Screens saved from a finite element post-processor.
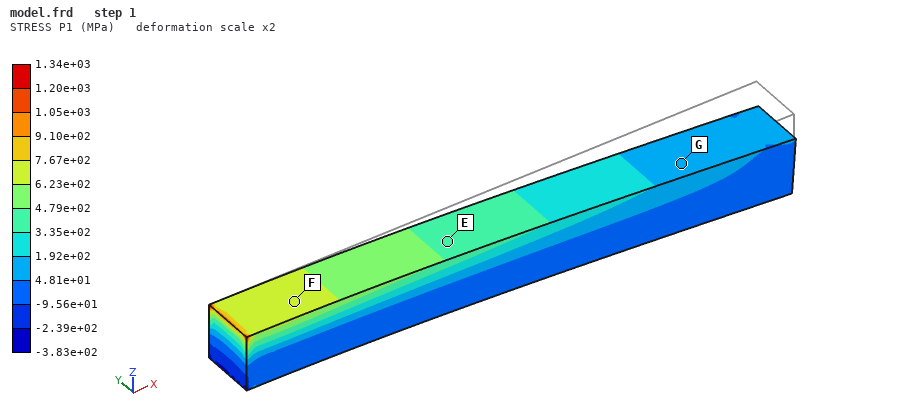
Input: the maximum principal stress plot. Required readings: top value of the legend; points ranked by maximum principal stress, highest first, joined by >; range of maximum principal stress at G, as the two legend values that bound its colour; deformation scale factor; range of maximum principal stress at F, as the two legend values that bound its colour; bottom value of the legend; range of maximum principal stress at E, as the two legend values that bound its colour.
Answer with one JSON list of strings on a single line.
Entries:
["1.34e+03 MPa", "F > E > G", "4.81e+01 to 1.92e+02 MPa", "2", "6.23e+02 to 7.67e+02 MPa", "-3.83e+02 MPa", "3.35e+02 to 4.79e+02 MPa"]
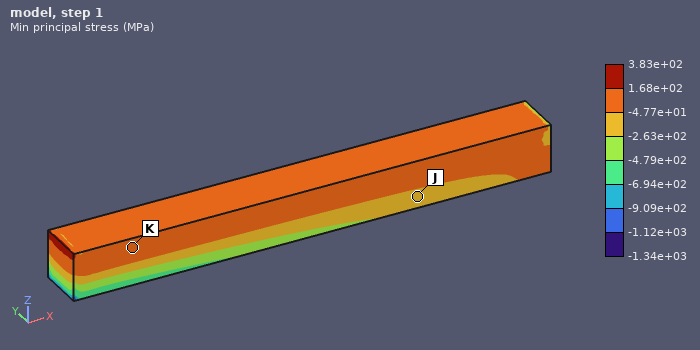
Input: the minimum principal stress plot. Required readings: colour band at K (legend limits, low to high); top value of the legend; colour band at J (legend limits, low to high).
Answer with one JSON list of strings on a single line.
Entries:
["-4.77e+01 to 1.68e+02 MPa", "3.83e+02 MPa", "-2.63e+02 to -4.77e+01 MPa"]
